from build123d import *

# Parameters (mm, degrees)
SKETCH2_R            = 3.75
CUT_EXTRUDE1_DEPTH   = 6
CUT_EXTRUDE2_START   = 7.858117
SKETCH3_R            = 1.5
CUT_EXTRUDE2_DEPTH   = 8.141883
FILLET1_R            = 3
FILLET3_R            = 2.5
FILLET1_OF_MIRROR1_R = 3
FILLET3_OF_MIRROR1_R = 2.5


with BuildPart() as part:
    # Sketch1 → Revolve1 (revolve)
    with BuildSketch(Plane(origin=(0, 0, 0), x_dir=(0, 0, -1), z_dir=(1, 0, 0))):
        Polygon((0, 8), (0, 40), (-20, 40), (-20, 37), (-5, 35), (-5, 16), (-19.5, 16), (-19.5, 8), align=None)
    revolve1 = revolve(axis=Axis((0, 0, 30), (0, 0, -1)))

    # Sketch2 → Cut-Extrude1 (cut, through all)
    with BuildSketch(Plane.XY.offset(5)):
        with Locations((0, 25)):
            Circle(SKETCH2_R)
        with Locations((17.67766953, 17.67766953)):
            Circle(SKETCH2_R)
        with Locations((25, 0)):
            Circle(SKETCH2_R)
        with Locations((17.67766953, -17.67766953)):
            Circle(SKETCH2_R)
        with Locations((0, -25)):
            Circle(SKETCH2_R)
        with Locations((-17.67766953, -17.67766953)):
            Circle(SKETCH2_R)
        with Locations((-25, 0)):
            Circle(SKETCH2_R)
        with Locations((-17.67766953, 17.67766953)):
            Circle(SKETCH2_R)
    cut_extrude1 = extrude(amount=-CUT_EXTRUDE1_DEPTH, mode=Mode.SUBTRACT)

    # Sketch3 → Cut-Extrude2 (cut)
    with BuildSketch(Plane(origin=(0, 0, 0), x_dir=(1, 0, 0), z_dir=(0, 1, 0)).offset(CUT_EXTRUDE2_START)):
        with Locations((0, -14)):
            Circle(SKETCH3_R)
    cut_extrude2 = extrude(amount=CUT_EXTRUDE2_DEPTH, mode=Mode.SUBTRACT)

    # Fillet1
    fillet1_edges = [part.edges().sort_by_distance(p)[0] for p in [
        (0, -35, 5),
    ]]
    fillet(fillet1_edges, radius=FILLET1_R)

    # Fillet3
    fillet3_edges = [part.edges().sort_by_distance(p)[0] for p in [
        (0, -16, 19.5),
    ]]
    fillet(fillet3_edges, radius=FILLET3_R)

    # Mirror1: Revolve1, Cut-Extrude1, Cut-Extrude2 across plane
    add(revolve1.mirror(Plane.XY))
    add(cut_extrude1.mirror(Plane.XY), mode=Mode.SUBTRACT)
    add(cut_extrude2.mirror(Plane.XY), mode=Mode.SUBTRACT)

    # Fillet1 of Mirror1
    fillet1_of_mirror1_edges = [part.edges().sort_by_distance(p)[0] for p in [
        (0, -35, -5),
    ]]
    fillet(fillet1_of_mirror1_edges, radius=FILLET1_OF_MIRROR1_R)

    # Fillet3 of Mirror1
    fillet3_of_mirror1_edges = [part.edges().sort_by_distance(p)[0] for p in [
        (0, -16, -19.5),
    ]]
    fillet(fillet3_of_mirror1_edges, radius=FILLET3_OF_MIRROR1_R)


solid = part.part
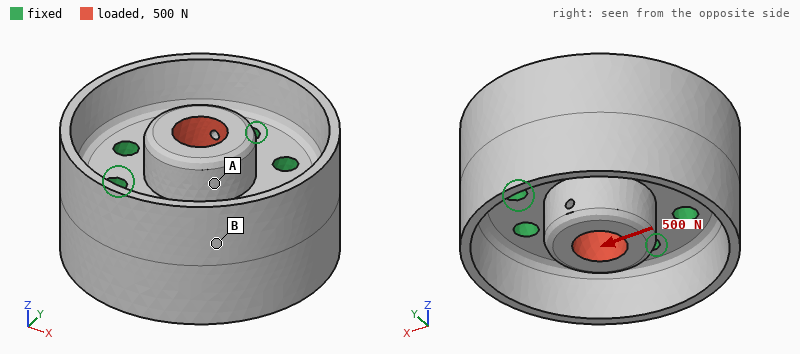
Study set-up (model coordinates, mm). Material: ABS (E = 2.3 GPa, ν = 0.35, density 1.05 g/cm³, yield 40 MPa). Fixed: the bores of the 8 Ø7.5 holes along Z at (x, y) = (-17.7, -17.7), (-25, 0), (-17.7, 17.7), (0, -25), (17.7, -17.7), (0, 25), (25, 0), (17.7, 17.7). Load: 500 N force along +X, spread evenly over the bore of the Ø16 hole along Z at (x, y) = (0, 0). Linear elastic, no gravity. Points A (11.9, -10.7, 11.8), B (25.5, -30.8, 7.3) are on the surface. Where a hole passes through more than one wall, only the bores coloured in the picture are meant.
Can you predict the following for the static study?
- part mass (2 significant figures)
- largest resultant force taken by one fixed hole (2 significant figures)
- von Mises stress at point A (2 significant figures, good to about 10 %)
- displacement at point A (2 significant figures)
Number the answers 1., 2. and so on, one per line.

1. 96 g
2. 100 N
3. 0.26 MPa
4. 5.8 µm
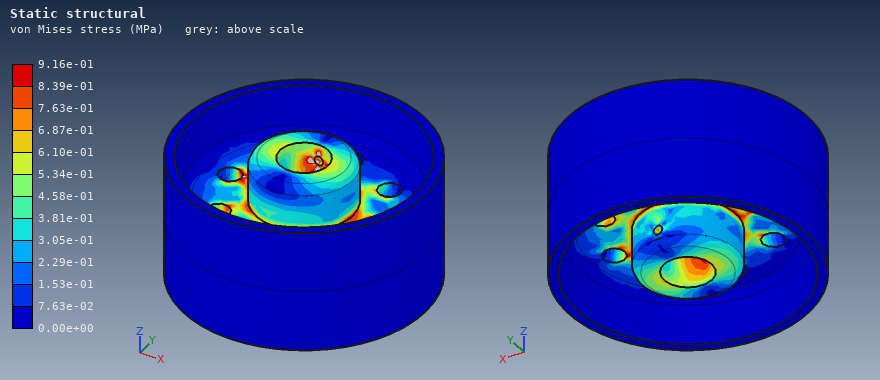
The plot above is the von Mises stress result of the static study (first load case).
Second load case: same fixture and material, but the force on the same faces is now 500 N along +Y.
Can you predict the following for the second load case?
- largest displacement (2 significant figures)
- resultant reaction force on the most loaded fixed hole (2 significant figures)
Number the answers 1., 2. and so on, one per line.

1. 10.0 µm
2. 100 N
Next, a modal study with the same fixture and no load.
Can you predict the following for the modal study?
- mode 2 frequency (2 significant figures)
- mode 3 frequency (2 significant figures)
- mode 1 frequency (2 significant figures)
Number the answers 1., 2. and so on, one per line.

1. 3700 Hz
2. 4100 Hz
3. 3700 Hz
